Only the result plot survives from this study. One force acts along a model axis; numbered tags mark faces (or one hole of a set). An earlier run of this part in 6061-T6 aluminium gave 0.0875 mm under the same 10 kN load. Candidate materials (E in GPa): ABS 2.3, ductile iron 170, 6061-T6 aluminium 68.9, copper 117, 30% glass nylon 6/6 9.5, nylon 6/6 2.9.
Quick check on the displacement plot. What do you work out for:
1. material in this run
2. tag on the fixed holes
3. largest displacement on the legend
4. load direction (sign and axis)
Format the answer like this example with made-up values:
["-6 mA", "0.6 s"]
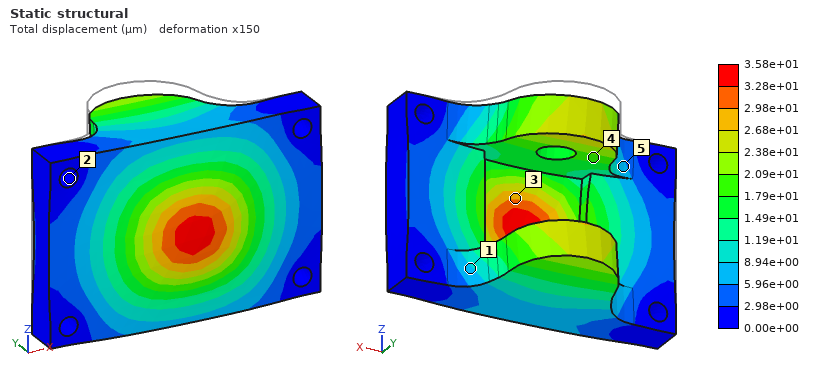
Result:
["ductile iron", "2", "3.58e+01 µm", "-Y"]
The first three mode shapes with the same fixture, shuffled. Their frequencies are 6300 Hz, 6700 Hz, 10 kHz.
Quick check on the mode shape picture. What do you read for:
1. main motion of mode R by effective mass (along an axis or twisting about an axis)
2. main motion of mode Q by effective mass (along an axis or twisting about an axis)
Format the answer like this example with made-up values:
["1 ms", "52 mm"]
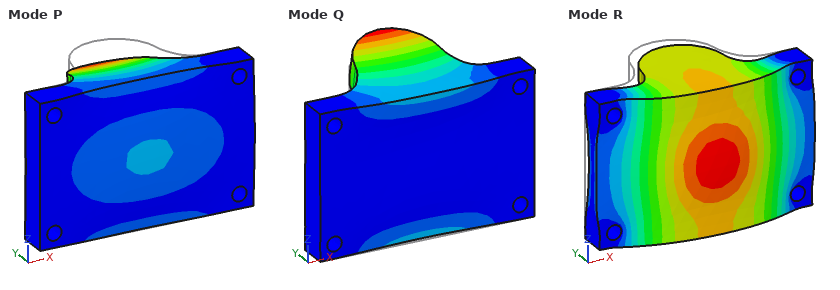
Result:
["along Y", "along Z"]
